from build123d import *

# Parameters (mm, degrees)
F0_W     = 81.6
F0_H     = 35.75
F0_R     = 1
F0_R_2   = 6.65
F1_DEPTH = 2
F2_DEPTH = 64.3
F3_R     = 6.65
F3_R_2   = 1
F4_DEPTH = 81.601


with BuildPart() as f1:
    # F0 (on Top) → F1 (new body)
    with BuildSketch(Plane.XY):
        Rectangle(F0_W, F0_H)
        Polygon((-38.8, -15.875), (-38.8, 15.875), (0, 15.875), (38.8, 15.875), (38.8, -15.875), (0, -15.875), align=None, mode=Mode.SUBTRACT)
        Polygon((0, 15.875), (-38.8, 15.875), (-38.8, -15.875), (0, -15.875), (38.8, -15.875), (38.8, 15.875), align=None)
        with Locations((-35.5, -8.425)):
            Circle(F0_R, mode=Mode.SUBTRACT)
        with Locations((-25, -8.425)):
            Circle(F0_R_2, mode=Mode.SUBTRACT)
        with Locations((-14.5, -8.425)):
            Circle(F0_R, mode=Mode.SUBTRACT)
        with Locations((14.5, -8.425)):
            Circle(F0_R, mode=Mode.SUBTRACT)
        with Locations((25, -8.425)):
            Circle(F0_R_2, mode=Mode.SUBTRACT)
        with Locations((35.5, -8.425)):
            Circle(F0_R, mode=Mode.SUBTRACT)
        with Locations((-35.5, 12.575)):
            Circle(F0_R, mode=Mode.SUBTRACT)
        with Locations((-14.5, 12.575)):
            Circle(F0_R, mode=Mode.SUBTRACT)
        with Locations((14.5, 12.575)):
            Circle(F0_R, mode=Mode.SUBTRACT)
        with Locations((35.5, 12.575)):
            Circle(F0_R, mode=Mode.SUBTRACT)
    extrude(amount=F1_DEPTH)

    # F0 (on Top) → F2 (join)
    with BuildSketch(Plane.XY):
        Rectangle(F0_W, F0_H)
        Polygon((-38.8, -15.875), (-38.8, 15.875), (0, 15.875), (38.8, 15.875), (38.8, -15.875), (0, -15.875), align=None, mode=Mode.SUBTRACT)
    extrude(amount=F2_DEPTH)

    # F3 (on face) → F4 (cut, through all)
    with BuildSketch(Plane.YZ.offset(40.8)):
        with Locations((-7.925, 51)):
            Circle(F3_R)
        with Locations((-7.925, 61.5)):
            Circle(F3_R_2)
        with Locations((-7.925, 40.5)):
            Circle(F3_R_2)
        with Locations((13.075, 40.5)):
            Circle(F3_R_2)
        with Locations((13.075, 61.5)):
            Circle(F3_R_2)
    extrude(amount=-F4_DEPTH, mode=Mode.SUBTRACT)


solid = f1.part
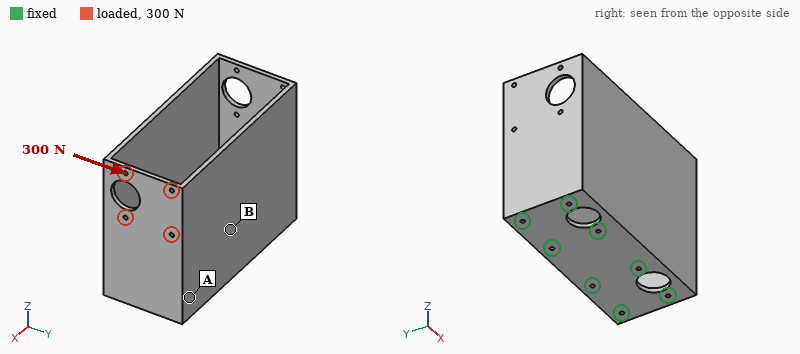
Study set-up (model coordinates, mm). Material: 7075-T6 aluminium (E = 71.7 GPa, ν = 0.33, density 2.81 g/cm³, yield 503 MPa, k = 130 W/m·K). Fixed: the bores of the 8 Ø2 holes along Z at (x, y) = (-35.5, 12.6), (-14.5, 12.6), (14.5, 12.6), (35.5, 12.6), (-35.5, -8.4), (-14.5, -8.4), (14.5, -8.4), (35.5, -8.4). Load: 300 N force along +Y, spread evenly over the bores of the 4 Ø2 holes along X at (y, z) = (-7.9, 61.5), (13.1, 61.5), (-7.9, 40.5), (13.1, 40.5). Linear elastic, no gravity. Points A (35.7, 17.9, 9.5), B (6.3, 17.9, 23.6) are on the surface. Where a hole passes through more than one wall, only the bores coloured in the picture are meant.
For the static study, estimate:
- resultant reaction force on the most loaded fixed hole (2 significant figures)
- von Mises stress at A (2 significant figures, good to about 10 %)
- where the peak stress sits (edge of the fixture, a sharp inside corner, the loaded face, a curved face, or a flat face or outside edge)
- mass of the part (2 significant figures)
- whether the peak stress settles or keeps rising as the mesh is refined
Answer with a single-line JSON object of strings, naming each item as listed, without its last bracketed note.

{"resultant reaction force on the most loaded fixed hole": "550 N", "von Mises stress at A": "12 MPa", "where the peak stress sits": "edge of the fixture", "mass of the part": "92 g", "whether the peak stress settles or keeps rising as the mesh is refined": "keeps rising"}
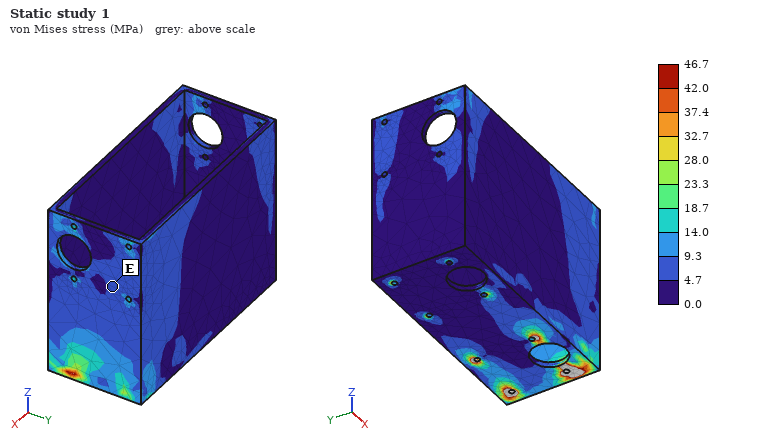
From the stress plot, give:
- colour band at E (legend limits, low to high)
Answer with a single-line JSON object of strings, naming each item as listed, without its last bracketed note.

{"colour band at E": "4.7 to 9.3 MPa"}
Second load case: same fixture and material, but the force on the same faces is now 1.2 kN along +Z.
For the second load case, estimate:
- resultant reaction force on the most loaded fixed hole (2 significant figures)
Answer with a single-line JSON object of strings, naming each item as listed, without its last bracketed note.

{"resultant reaction force on the most loaded fixed hole": "550 N"}
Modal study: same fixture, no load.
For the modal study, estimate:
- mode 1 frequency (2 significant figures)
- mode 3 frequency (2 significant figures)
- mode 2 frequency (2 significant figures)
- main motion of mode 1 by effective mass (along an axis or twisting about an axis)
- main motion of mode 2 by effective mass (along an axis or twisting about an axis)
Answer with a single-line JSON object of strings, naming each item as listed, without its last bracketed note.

{"mode 1 frequency": "1300 Hz", "mode 3 frequency": "2200 Hz", "mode 2 frequency": "1400 Hz", "main motion of mode 1 by effective mass": "along Y", "main motion of mode 2 by effective mass": "along Y"}
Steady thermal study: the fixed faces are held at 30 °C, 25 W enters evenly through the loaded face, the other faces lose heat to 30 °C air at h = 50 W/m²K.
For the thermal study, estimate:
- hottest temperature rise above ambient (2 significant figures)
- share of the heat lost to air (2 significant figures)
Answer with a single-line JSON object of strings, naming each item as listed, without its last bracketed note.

{"hottest temperature rise above ambient": "49 K", "share of the heat lost to air": "53 %"}
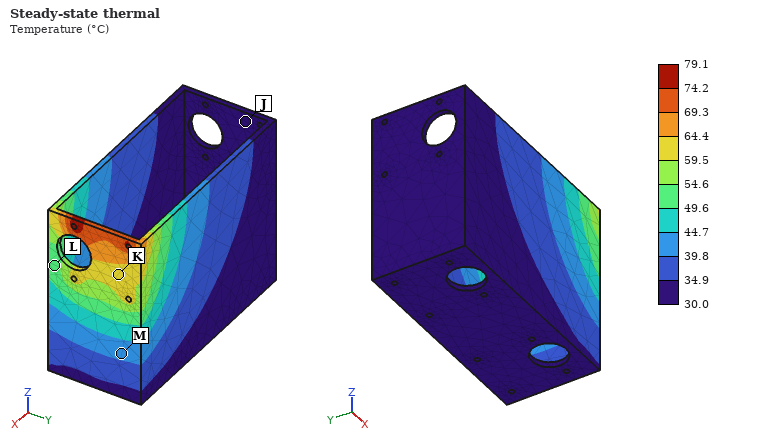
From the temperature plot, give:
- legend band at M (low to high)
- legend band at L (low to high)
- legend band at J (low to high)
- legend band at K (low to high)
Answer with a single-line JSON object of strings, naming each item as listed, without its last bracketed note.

{"legend band at M": "39.8 to 44.7 °C", "legend band at L": "49.6 to 54.6 °C", "legend band at J": "30.0 to 34.9 °C", "legend band at K": "59.5 to 64.4 °C"}
